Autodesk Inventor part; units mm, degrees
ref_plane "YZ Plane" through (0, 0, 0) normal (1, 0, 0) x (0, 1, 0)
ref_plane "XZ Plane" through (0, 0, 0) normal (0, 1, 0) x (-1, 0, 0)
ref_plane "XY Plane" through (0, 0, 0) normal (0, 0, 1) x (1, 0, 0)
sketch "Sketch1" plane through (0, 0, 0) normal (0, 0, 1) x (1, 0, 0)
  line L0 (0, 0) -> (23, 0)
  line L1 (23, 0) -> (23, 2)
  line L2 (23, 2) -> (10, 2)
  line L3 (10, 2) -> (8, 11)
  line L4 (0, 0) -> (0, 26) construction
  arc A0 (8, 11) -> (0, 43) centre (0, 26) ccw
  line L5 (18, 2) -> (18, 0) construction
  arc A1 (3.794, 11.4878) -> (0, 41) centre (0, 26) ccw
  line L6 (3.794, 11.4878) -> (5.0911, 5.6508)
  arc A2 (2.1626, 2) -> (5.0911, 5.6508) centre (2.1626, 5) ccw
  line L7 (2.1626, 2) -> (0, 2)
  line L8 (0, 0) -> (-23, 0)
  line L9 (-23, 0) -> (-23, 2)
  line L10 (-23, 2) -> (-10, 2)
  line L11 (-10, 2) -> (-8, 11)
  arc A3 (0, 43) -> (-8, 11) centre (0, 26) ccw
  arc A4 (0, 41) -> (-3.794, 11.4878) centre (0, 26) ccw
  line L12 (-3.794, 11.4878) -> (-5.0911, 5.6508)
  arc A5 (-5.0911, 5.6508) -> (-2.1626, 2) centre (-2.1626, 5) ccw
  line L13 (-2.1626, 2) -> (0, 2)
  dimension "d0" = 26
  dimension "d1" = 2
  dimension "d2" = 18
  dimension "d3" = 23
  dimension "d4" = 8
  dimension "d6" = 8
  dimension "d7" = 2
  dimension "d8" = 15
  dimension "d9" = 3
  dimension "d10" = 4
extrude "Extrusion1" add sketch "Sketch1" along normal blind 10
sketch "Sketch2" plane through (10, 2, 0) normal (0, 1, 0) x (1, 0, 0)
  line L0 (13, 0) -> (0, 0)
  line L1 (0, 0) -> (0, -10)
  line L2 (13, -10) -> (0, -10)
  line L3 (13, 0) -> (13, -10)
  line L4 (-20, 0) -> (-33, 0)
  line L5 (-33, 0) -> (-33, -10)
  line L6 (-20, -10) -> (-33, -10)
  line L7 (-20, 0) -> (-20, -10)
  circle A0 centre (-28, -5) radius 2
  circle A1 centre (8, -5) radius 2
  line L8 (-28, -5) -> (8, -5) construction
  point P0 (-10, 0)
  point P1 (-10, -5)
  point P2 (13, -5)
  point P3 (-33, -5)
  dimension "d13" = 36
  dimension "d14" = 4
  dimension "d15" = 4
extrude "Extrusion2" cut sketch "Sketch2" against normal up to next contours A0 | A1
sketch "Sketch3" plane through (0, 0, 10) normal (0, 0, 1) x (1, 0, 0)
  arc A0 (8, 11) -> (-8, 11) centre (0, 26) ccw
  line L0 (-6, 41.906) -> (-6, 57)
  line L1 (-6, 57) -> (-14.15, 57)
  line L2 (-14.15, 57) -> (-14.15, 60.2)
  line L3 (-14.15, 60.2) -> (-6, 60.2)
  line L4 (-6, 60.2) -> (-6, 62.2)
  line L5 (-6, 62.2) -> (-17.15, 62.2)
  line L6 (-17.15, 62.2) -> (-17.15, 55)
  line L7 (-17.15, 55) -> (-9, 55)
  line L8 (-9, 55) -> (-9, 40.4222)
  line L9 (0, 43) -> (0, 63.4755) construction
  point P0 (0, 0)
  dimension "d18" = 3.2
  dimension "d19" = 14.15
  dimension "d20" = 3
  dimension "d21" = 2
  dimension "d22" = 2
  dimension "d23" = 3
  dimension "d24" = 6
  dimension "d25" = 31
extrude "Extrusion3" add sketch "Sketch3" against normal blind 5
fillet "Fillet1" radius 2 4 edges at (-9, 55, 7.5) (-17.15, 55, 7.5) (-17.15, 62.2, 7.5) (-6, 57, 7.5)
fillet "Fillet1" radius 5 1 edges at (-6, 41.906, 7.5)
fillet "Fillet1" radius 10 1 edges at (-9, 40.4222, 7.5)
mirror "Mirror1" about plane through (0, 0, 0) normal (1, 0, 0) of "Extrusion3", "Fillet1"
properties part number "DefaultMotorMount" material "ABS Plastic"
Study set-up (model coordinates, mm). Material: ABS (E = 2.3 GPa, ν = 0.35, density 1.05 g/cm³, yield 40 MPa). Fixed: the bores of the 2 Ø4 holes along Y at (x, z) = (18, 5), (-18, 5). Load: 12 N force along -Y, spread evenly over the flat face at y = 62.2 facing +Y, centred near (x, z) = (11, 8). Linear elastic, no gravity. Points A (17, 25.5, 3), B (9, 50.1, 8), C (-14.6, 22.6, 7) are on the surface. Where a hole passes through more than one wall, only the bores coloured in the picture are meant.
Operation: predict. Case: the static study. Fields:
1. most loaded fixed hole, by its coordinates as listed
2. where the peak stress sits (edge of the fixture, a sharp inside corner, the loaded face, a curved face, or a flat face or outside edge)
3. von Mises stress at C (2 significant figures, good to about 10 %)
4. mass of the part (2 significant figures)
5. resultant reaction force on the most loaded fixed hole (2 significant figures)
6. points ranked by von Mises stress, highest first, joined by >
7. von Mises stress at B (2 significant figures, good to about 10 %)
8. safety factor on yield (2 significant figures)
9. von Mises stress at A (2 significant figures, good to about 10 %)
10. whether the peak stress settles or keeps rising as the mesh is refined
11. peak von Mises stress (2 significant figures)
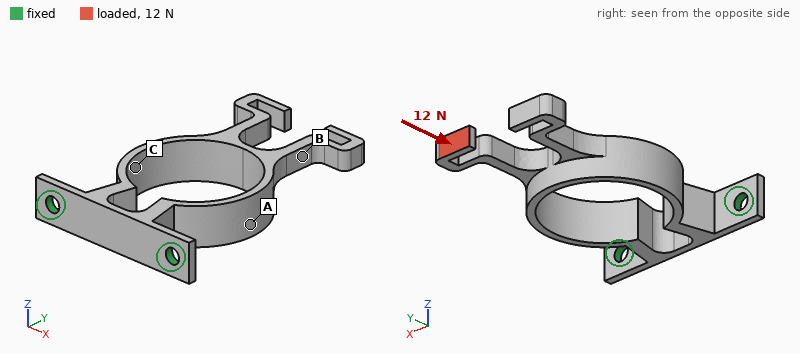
(18, 5)
the loaded face
1.7 MPa
4.7 g
11 N
B > A > C
5.7 MPa
3.4
3.6 MPa
settles
12 MPa
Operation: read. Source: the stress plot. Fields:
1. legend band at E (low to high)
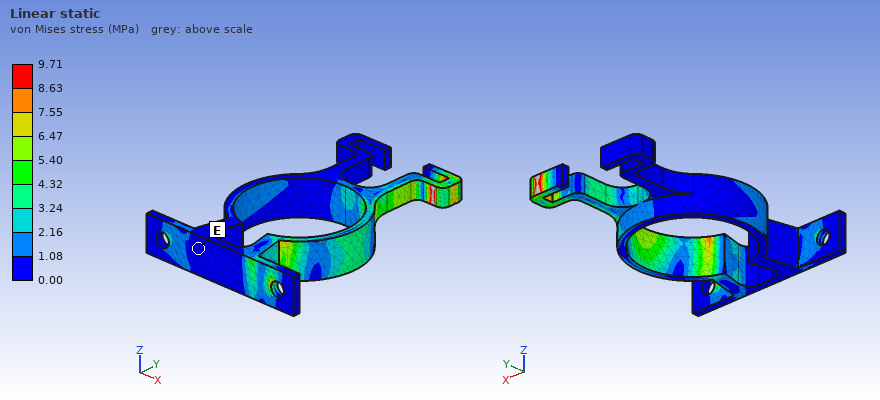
0.00 to 1.08 MPa
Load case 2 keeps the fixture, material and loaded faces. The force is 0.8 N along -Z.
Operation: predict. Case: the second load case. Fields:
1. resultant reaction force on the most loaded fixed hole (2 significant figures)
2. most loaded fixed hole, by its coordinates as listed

0.69 N
(18, 5)
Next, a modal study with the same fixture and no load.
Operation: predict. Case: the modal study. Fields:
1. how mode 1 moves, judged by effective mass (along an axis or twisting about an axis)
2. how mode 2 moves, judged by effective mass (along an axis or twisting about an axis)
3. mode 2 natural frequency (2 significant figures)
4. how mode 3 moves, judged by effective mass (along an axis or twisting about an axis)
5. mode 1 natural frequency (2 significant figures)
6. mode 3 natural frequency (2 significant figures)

along Z
along X
260 Hz
twisting about Y
170 Hz
640 Hz
